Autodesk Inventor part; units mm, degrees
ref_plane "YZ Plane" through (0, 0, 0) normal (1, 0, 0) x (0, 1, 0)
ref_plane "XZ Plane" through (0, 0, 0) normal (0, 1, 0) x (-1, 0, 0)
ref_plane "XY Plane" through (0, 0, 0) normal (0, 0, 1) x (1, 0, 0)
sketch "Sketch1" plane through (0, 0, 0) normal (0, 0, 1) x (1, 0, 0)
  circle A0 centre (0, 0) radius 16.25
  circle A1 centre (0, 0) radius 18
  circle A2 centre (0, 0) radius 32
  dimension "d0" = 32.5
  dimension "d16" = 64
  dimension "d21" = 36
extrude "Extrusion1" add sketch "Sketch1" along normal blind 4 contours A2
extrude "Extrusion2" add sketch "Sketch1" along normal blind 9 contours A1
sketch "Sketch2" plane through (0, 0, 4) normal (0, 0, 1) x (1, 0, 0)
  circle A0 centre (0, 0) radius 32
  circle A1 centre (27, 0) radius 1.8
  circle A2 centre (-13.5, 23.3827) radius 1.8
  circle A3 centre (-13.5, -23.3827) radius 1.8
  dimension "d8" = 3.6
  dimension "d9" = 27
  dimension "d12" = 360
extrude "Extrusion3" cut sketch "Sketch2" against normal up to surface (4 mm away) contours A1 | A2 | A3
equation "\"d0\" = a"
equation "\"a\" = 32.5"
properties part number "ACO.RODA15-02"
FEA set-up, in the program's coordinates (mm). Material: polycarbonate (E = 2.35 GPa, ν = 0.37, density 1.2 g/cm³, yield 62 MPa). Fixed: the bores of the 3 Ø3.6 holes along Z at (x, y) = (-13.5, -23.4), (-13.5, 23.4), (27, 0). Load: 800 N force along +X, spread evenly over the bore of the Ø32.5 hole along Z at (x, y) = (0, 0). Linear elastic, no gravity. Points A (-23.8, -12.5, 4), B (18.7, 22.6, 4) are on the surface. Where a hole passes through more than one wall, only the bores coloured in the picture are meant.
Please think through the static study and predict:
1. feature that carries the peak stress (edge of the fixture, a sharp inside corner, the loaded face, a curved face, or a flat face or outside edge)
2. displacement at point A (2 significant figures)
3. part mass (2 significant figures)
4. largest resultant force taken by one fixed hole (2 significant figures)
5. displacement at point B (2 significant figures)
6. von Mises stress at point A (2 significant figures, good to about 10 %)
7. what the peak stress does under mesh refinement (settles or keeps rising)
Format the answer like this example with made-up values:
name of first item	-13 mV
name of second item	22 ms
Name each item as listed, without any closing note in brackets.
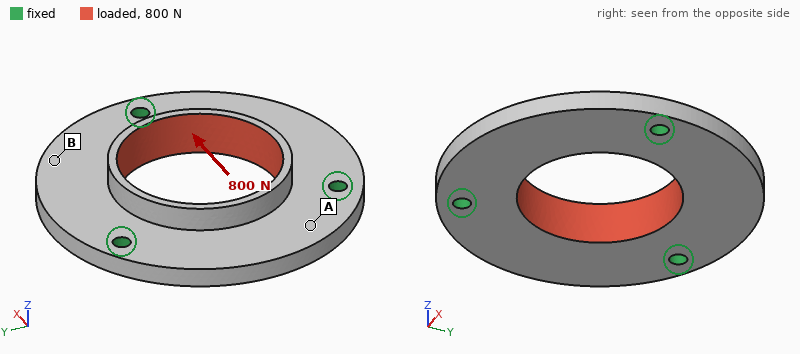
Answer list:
feature that carries the peak stress	edge of the fixture
displacement at point A	0.096 mm
part mass	12 g
largest resultant force taken by one fixed hole	310 N
displacement at point B	0.080 mm
von Mises stress at point A	3.0 MPa
what the peak stress does under mesh refinement	keeps rising
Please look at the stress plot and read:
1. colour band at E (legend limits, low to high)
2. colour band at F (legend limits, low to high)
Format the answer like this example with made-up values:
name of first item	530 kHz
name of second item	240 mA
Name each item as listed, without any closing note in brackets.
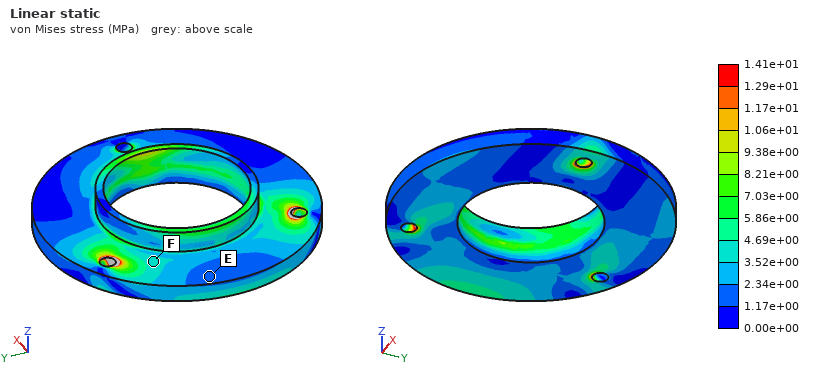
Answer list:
colour band at E	1.17e+00 to 2.34e+00 MPa
colour band at F	3.52e+00 to 4.69e+00 MPa
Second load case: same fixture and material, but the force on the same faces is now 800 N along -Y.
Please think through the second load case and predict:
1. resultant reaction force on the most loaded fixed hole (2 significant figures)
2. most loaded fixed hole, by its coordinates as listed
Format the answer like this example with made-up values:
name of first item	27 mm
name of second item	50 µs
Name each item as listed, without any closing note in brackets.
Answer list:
resultant reaction force on the most loaded fixed hole	330 N
most loaded fixed hole, by its coordinates as listed	(27, 0)
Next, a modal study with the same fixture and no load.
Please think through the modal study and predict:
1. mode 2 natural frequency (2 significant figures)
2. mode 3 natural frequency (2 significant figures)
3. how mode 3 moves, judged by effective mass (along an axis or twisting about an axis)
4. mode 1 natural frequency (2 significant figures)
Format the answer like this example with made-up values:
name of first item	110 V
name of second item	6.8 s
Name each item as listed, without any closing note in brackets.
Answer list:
mode 2 natural frequency	1700 Hz
mode 3 natural frequency	2100 Hz
how mode 3 moves, judged by effective mass	along Z
mode 1 natural frequency	1700 Hz
